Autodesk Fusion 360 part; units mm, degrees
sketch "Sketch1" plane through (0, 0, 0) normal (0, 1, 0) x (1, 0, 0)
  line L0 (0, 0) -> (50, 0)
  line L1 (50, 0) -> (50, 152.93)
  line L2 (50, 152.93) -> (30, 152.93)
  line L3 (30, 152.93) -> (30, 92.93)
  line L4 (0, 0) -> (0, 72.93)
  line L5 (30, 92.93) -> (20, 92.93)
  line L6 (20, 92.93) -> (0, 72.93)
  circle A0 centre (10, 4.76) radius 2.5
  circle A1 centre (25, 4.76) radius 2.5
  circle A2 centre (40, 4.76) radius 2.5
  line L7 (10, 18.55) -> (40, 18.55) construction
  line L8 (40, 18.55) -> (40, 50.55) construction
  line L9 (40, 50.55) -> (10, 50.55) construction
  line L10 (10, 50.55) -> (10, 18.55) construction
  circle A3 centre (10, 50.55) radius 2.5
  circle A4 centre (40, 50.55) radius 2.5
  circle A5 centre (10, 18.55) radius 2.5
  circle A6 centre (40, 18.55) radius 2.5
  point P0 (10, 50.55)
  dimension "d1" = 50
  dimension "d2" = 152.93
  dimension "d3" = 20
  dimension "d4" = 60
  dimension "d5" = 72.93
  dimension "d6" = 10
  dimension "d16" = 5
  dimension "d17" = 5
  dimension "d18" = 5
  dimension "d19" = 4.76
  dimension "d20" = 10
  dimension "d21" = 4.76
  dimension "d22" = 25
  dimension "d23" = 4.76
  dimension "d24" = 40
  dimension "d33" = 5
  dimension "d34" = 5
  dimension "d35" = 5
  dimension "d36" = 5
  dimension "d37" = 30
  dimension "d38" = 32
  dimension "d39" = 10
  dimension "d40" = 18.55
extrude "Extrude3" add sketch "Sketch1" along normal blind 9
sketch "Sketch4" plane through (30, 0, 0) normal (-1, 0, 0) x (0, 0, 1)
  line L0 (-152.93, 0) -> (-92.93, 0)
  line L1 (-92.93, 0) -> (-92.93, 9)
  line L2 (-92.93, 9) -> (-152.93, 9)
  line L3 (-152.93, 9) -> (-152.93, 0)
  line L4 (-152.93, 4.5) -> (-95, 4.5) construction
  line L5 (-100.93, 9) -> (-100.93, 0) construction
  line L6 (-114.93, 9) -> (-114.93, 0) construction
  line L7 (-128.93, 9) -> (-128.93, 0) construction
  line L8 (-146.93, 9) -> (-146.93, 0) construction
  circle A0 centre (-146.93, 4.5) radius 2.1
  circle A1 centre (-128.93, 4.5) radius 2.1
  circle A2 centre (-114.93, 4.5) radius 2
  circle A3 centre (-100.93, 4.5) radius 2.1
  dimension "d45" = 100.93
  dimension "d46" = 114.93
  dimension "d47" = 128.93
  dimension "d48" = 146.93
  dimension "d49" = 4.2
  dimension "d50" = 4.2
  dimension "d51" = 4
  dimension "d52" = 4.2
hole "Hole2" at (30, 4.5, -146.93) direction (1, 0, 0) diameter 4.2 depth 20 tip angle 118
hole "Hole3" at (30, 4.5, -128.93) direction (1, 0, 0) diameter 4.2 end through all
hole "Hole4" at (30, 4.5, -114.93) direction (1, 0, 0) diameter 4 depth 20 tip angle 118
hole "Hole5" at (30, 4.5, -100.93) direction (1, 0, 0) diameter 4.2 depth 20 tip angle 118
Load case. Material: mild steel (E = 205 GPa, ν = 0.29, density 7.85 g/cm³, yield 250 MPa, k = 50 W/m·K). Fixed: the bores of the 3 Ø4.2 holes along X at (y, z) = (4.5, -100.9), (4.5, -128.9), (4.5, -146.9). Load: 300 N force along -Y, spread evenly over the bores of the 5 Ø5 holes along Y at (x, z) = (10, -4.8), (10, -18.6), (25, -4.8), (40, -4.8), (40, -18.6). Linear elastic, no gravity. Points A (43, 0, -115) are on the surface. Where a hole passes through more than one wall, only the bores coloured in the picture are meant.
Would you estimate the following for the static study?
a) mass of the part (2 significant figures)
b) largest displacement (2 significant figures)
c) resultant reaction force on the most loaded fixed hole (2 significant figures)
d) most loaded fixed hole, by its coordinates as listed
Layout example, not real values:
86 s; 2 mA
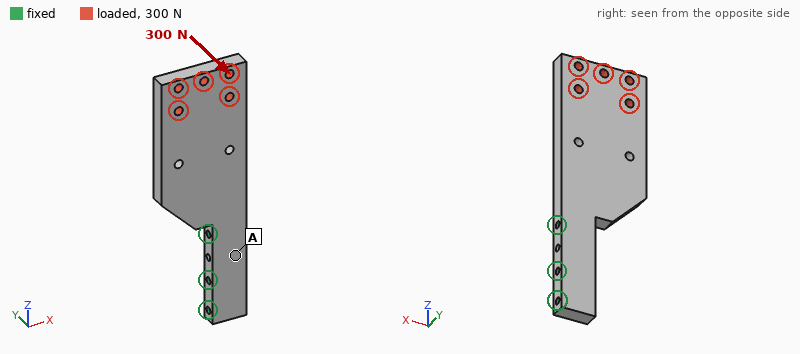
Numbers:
380 g; 0.27 mm; 480 N; (4.5, -100.9)
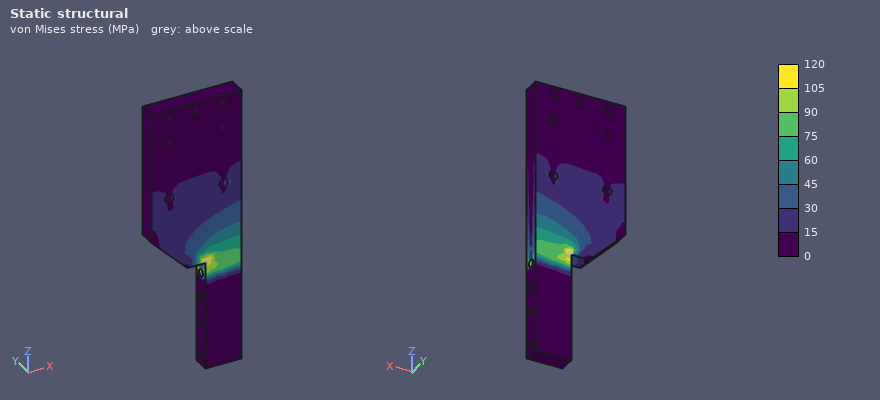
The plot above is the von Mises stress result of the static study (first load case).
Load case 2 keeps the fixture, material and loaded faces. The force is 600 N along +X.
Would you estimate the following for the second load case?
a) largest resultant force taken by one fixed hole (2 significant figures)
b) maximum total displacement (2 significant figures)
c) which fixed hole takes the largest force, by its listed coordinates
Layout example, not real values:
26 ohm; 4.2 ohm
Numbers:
660 N; 78 µm; (4.5, -100.9)
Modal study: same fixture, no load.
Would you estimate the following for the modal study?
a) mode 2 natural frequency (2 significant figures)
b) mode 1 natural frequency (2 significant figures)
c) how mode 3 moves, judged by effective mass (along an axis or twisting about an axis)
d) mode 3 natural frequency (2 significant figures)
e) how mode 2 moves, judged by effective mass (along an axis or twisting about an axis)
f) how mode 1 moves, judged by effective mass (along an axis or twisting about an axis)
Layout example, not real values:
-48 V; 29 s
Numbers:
1300 Hz; 520 Hz; twisting about Z; 2000 Hz; along X; along Y
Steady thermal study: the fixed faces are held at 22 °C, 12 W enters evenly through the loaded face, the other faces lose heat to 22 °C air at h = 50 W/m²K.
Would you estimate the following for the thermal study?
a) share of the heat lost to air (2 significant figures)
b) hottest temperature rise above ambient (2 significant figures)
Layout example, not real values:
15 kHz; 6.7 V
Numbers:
73 %; 28 K
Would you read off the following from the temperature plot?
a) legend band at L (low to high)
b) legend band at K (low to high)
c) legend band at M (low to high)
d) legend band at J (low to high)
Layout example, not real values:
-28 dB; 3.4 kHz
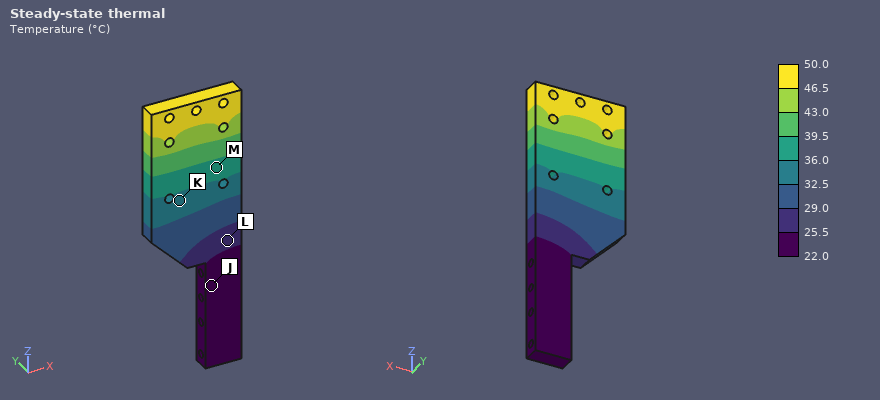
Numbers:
25.5 to 29.0 °C; 32.5 to 36.0 °C; 36.0 to 39.5 °C; 22.0 to 25.5 °C
